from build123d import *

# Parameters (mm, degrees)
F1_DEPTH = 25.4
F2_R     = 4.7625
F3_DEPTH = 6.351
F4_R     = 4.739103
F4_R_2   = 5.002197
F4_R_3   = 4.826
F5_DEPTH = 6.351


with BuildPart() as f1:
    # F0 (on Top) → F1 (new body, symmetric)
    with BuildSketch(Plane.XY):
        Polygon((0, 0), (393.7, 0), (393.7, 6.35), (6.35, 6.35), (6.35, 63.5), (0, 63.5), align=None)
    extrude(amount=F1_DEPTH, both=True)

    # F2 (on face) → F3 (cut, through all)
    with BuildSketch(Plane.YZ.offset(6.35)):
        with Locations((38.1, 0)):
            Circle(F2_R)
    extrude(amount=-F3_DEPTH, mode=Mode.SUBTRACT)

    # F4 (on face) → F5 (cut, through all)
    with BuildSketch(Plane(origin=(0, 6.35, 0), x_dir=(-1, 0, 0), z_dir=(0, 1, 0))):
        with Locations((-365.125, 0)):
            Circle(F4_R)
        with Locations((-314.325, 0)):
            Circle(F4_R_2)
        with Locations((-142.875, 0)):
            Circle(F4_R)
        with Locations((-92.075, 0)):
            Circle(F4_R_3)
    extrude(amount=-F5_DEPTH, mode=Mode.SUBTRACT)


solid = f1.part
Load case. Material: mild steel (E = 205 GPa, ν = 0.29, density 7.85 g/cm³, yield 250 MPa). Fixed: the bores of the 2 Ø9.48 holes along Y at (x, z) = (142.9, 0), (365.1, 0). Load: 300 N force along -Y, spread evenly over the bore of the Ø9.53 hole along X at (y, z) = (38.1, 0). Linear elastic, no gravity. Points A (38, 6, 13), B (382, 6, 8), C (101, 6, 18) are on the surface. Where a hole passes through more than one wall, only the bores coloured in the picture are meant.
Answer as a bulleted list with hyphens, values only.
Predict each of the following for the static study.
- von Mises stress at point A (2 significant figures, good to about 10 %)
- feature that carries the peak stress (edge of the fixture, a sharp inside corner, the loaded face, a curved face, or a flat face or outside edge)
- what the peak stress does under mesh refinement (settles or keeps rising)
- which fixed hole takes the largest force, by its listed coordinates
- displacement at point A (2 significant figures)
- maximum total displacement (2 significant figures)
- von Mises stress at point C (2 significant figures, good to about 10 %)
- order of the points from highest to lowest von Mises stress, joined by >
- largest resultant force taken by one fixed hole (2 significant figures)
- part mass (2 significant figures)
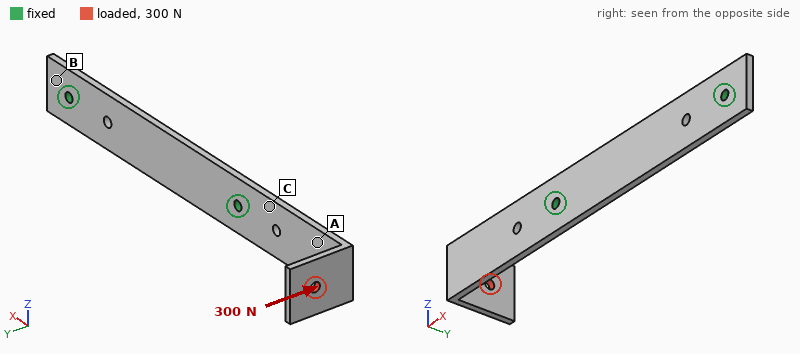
- 31 MPa
- edge of the fixture
- keeps rising
- (142.9, 0)
- 0.77 mm
- 1.5 mm
- 92 MPa
- C > A > B
- 310 N
- 1.1 kg
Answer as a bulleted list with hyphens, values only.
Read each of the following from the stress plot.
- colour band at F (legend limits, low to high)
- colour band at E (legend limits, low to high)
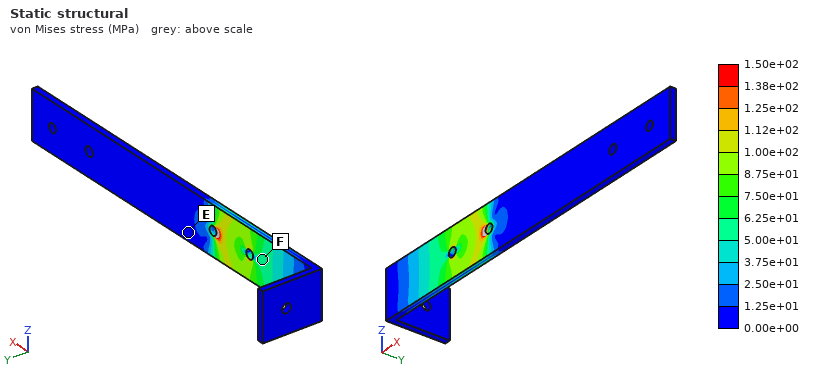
- 5.00e+01 to 6.25e+01 MPa
- 0.00e+00 to 1.25e+01 MPa
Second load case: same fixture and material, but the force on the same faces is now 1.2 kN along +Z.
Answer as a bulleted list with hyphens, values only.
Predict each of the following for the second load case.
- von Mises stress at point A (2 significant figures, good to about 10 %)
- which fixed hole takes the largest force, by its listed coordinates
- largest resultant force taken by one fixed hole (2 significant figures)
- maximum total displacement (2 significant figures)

- 120 MPa
- (142.9, 0)
- 1.7 kN
- 1.3 mm
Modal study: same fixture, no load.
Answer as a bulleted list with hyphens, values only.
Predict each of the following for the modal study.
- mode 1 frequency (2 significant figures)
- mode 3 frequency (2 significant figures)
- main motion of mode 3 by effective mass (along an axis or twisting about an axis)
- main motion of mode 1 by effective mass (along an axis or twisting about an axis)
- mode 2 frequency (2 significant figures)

- 160 Hz
- 680 Hz
- along Y
- along Y
- 470 Hz
